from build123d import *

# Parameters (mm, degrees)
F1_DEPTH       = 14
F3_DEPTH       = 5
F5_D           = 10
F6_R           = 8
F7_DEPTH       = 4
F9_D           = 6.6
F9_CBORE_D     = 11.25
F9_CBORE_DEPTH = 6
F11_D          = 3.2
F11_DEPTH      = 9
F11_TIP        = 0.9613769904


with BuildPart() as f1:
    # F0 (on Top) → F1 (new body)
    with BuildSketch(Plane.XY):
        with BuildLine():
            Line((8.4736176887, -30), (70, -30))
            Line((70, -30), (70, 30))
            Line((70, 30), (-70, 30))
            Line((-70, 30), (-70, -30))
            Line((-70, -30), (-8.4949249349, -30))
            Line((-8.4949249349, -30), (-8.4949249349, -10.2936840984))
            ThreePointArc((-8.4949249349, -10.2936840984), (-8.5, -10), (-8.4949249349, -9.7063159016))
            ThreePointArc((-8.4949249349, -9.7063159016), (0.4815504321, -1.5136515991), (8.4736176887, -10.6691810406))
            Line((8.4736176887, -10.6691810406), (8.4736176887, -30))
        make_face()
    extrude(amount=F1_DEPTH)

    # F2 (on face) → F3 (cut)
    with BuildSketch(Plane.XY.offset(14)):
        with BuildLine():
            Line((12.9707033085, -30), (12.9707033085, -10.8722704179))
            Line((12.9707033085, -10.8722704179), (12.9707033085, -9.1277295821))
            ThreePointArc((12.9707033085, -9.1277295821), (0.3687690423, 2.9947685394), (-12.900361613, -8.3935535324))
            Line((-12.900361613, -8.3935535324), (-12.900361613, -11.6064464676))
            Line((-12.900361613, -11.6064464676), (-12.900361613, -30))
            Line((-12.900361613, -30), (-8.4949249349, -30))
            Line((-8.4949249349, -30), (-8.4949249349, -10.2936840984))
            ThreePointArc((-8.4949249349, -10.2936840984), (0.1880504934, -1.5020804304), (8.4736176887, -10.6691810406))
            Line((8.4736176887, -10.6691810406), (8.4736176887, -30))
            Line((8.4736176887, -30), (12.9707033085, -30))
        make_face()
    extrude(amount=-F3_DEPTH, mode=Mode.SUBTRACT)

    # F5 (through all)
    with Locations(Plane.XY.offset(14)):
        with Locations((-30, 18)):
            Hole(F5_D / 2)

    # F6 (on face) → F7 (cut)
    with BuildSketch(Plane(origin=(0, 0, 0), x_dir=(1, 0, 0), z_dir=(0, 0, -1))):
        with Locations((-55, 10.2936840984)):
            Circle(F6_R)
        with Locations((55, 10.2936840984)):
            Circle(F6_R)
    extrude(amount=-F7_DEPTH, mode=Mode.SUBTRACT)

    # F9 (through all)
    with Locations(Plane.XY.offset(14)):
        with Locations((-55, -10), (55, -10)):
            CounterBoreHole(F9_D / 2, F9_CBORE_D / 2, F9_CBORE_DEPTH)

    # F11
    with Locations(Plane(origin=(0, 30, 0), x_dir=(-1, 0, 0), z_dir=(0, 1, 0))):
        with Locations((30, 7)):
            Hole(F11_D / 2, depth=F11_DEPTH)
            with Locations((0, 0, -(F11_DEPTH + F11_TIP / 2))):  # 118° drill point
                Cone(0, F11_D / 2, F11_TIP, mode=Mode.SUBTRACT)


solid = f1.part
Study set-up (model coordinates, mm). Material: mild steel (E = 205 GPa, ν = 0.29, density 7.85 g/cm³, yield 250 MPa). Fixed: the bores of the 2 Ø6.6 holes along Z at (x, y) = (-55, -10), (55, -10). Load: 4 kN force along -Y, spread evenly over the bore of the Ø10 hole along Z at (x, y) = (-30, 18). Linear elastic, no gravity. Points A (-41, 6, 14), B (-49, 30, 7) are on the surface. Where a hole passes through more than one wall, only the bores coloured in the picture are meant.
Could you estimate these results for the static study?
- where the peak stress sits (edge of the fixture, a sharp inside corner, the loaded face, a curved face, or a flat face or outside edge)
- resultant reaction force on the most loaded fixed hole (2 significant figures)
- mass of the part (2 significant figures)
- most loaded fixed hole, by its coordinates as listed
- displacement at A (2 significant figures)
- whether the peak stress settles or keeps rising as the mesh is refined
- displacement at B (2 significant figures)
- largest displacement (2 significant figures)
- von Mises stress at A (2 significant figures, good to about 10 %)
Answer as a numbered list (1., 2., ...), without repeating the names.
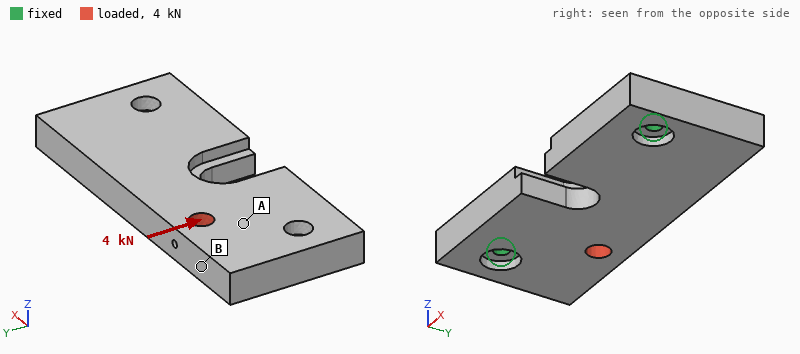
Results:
1. edge of the fixture
2. 3.4 kN
3. 830 g
4. (-55, -10)
5. 4.2 µm
6. keeps rising
7. 5.4 µm
8. 7.4 µm
9. 9.4 MPa
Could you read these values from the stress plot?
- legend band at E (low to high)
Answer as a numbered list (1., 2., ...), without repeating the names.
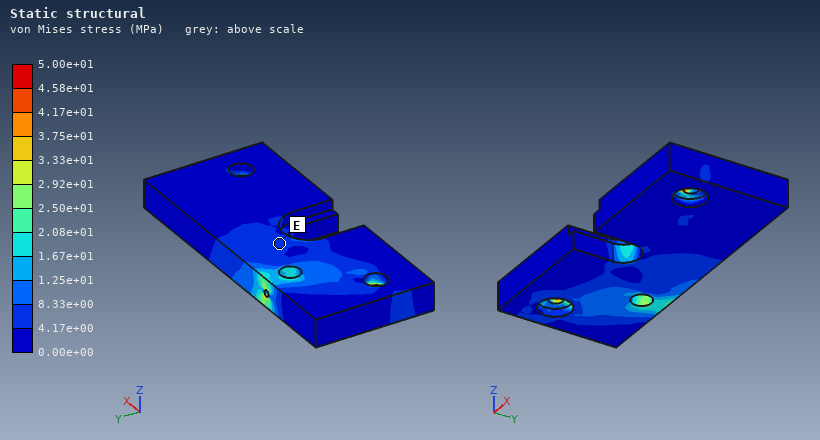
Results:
1. 4.17e+00 to 8.33e+00 MPa
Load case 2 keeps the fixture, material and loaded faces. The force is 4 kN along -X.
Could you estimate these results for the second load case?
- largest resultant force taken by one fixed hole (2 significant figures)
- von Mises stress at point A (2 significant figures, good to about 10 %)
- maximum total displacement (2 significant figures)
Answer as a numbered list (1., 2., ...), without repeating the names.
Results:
1. 2.3 kN
2. 5.1 MPa
3. 3.8 µm
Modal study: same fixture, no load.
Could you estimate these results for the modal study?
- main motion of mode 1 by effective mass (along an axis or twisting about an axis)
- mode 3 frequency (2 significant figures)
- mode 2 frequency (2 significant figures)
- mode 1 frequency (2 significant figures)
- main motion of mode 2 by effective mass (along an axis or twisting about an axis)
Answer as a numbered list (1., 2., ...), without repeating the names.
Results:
1. along Z
2. 3800 Hz
3. 3000 Hz
4. 1600 Hz
5. along Z
